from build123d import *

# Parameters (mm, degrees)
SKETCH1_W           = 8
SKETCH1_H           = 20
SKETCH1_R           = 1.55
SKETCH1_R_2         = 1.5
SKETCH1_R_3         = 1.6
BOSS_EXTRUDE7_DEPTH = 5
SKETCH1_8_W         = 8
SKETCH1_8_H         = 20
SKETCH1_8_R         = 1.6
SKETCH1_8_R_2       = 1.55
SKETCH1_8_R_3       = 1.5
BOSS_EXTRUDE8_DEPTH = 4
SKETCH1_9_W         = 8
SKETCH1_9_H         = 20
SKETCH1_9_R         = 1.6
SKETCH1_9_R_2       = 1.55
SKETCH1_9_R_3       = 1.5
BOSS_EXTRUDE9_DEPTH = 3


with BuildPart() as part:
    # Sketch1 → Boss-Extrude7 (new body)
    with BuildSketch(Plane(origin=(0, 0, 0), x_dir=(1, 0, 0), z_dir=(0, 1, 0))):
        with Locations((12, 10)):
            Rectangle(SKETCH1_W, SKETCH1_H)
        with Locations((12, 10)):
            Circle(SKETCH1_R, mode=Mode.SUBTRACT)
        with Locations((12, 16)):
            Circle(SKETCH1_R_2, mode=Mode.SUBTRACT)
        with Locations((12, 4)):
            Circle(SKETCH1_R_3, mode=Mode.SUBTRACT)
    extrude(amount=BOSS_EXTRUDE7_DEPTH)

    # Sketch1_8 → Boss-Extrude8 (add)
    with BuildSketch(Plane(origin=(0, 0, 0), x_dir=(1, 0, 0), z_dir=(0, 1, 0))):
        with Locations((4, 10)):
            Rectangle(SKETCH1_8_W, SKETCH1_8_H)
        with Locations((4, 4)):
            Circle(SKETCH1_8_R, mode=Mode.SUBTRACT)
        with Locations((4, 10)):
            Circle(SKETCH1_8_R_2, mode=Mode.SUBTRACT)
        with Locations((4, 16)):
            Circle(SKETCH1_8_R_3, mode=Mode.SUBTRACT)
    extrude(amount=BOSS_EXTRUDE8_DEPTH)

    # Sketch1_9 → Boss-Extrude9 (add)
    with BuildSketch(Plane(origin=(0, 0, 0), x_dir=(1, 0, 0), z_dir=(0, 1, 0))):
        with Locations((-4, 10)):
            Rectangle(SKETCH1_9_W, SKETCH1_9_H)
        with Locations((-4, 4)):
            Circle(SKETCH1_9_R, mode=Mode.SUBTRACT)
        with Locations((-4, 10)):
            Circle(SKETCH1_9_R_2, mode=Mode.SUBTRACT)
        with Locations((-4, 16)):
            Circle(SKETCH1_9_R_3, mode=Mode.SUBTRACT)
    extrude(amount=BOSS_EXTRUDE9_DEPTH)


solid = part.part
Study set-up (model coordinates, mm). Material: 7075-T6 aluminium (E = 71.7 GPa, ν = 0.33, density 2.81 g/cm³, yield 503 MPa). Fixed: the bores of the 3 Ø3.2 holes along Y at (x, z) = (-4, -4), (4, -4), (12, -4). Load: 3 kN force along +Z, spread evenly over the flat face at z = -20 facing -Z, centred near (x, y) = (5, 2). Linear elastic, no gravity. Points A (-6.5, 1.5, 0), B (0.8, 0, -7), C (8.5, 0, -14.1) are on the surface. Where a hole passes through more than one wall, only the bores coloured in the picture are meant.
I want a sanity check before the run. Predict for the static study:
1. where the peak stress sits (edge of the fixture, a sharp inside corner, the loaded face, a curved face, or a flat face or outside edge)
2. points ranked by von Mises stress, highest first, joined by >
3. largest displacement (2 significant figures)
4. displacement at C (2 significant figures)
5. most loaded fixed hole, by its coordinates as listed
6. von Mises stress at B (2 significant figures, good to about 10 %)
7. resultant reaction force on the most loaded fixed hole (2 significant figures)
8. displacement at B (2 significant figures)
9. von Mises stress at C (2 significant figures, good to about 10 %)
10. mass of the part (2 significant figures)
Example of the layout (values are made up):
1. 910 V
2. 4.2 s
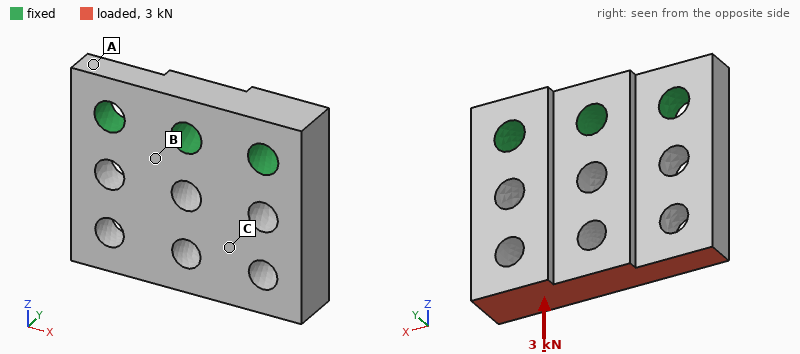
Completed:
1. a curved face
2. C > B > A
3. 10 µm
4. 5.8 µm
5. (12, -4)
6. 29 MPa
7. 1.3 kN
8. 1.6 µm
9. 51 MPa
10. 4.6 g
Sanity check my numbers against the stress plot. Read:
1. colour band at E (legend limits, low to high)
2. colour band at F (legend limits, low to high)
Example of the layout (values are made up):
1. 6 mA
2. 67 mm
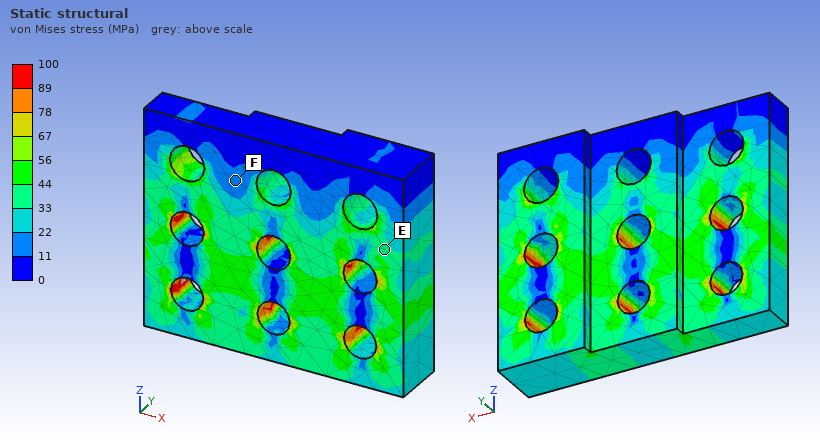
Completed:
1. 33 to 44 MPa
2. 11 to 22 MPa
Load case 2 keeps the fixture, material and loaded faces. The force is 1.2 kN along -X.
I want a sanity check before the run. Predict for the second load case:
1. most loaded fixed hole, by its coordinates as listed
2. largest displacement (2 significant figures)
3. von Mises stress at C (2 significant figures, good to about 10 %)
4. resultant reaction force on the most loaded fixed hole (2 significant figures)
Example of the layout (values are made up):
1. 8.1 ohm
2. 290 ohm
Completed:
1. (12, -4)
2. 27 µm
3. 24 MPa
4. 1.2 kN
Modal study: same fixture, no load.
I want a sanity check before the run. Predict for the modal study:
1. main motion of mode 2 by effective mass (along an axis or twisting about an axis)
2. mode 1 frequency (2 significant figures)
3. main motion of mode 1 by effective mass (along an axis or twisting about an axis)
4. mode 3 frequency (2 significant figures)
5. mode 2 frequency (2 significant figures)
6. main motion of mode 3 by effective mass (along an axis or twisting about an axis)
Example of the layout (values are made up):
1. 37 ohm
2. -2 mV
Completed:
1. twisting about Z
2. 13 kHz
3. along Y
4. 34 kHz
5. 20 kHz
6. along X
